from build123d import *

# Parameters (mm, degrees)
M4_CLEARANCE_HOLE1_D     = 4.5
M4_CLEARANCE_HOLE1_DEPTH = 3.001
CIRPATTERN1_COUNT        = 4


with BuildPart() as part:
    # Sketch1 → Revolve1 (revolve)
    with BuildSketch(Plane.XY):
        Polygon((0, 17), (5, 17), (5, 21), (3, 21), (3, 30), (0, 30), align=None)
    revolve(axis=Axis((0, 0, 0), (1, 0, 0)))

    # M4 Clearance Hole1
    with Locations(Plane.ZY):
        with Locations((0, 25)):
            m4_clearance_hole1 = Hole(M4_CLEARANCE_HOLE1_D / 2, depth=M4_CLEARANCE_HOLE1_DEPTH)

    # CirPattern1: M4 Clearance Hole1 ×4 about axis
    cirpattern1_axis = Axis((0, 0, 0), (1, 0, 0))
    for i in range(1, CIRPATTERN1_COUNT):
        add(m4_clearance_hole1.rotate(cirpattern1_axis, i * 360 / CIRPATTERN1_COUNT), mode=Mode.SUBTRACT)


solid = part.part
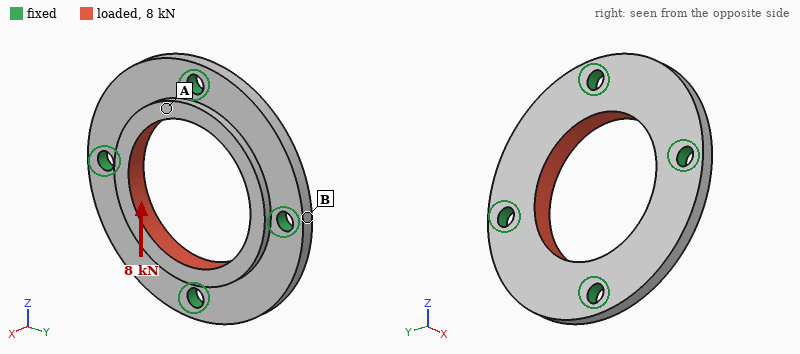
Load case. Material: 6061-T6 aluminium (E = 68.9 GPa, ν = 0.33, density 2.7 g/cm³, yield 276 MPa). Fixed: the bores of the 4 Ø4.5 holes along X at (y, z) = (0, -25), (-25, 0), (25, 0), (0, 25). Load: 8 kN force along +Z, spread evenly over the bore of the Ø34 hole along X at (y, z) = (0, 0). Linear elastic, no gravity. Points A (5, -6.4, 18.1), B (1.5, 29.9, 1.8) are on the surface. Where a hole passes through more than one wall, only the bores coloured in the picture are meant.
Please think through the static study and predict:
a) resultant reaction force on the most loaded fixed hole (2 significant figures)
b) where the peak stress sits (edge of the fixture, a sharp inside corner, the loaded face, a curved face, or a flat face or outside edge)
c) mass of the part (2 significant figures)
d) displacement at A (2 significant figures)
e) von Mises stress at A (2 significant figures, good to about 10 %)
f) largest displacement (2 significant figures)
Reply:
2.3 kN
edge of the fixture
18 g
12 µm
37 MPa
18 µm
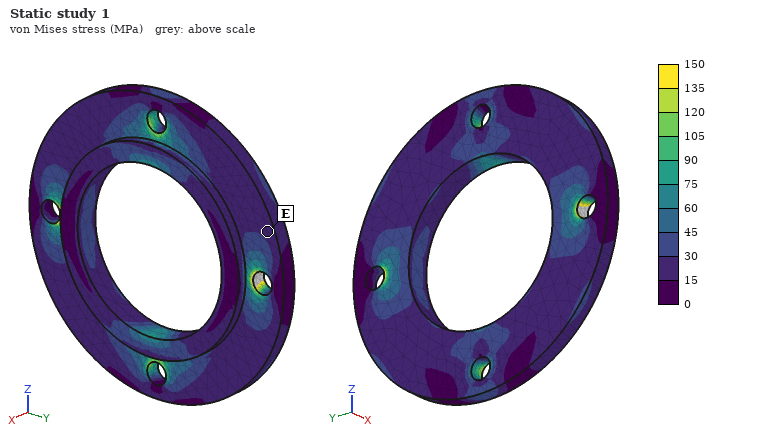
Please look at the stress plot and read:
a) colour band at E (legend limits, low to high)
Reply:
15 to 30 MPa
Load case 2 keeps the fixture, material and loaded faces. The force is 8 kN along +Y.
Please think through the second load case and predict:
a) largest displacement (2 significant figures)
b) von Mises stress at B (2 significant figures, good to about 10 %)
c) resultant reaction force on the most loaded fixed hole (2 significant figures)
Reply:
18 µm
35 MPa
2.3 kN
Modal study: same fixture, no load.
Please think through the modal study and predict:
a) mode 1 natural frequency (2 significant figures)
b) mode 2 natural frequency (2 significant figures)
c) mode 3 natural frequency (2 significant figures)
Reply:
11 kHz
12 kHz
12 kHz
